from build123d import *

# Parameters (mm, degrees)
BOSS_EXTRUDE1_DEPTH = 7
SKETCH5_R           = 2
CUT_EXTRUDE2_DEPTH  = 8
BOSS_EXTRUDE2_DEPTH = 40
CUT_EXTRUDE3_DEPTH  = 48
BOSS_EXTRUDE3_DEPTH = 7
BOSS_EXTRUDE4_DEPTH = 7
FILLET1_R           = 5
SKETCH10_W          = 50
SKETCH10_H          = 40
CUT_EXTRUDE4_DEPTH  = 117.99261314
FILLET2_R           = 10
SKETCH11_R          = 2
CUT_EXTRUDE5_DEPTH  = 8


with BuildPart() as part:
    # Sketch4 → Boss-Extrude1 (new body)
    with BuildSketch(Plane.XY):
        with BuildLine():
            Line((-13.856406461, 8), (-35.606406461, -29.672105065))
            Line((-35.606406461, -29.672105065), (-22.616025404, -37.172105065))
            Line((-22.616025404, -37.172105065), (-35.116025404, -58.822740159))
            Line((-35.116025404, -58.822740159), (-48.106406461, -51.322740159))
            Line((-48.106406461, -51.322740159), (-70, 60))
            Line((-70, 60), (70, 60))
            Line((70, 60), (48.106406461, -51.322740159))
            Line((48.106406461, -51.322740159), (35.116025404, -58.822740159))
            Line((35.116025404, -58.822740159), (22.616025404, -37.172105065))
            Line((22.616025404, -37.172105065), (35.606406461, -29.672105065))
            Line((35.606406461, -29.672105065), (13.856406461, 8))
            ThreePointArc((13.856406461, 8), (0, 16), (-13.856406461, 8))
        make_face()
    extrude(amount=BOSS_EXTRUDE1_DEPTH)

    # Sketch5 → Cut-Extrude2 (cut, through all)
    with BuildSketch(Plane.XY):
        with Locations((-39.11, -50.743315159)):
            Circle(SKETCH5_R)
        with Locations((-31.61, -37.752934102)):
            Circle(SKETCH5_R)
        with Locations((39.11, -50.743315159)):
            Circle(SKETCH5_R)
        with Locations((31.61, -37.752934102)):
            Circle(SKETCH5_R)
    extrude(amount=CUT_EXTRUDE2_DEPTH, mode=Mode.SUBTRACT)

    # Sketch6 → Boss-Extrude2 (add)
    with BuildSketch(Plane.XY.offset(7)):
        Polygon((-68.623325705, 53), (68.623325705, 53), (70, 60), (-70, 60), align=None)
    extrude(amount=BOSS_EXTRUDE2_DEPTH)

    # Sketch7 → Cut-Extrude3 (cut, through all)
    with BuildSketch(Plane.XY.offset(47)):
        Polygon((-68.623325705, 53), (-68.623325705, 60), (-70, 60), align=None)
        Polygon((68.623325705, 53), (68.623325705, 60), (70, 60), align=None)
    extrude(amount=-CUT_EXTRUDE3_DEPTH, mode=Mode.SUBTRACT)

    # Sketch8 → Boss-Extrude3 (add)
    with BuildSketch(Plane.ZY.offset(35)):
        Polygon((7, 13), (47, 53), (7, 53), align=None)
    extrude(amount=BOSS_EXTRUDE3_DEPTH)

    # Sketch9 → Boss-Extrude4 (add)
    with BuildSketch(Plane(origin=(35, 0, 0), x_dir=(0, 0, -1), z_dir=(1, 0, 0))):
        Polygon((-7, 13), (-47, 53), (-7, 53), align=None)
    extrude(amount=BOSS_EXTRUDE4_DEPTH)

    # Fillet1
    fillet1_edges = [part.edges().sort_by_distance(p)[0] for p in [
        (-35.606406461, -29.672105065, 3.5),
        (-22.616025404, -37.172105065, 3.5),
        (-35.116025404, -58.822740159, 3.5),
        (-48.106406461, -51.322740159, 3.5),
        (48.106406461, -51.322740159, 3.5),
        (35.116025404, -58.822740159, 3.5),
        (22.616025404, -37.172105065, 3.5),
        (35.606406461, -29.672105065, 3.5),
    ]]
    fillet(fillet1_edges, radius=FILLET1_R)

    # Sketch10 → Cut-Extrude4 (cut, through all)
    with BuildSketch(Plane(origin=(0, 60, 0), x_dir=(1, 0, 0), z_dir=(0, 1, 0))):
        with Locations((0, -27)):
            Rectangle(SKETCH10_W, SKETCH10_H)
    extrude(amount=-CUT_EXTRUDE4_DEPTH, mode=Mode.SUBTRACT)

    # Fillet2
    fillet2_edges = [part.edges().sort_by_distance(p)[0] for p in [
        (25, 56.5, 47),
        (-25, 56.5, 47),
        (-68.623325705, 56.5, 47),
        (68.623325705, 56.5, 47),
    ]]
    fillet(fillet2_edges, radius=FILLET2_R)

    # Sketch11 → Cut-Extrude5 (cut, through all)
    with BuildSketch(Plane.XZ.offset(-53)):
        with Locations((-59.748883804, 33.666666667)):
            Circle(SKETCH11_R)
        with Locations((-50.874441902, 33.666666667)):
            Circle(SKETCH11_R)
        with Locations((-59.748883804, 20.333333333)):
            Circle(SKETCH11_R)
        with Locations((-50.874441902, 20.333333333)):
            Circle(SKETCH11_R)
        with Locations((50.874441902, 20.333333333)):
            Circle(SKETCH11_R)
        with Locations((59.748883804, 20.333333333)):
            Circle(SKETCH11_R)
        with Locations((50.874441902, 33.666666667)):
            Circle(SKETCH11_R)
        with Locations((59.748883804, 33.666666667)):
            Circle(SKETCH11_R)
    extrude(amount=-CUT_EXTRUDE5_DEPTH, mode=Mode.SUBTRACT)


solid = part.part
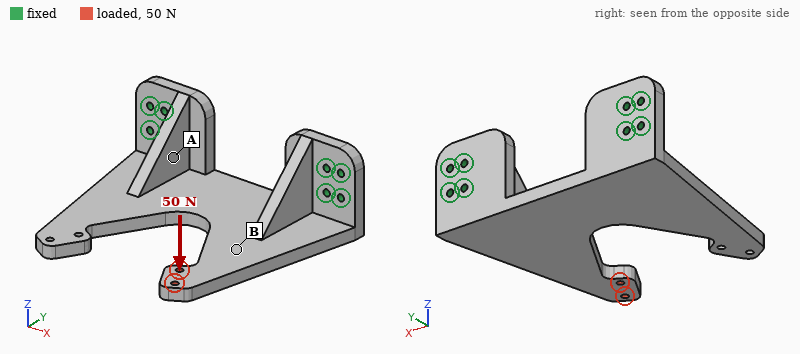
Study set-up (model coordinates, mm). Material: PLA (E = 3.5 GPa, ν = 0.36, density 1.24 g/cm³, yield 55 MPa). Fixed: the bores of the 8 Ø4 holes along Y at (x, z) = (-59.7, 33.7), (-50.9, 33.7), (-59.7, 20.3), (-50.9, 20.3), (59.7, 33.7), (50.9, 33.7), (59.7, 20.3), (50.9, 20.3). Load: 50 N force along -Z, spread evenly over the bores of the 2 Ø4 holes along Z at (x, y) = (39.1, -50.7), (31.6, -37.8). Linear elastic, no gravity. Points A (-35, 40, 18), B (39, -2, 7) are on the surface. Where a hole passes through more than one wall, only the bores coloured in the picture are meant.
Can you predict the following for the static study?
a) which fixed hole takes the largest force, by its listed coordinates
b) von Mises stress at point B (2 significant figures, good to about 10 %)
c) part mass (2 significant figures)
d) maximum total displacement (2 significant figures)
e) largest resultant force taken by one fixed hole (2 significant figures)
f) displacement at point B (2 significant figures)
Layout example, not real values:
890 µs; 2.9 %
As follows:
(50.9, 33.7); 6.8 MPa; 130 g; 2.1 mm; 190 N; 0.42 mm
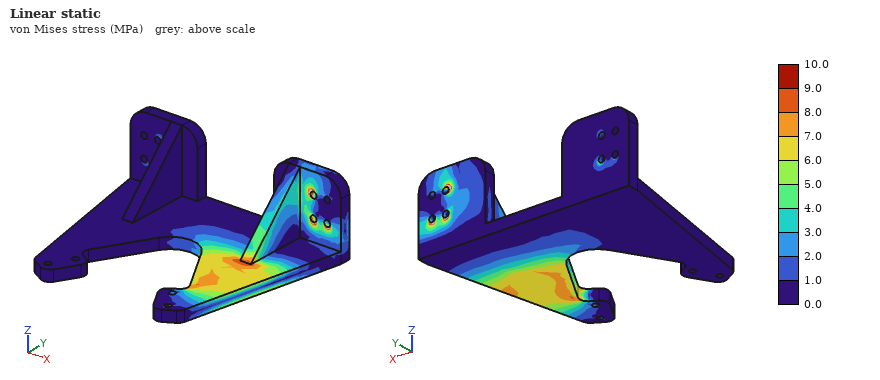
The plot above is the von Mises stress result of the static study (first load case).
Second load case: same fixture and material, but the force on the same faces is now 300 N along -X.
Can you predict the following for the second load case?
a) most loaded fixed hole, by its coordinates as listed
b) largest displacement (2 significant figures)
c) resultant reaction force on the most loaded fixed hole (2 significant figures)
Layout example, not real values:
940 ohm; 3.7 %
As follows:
(-50.9, 20.3); 0.93 mm; 350 N
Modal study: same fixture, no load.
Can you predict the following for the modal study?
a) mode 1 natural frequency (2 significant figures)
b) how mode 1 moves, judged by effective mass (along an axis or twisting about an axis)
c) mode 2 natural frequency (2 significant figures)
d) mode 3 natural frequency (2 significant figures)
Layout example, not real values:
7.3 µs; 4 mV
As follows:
340 Hz; along Z; 370 Hz; 910 Hz
